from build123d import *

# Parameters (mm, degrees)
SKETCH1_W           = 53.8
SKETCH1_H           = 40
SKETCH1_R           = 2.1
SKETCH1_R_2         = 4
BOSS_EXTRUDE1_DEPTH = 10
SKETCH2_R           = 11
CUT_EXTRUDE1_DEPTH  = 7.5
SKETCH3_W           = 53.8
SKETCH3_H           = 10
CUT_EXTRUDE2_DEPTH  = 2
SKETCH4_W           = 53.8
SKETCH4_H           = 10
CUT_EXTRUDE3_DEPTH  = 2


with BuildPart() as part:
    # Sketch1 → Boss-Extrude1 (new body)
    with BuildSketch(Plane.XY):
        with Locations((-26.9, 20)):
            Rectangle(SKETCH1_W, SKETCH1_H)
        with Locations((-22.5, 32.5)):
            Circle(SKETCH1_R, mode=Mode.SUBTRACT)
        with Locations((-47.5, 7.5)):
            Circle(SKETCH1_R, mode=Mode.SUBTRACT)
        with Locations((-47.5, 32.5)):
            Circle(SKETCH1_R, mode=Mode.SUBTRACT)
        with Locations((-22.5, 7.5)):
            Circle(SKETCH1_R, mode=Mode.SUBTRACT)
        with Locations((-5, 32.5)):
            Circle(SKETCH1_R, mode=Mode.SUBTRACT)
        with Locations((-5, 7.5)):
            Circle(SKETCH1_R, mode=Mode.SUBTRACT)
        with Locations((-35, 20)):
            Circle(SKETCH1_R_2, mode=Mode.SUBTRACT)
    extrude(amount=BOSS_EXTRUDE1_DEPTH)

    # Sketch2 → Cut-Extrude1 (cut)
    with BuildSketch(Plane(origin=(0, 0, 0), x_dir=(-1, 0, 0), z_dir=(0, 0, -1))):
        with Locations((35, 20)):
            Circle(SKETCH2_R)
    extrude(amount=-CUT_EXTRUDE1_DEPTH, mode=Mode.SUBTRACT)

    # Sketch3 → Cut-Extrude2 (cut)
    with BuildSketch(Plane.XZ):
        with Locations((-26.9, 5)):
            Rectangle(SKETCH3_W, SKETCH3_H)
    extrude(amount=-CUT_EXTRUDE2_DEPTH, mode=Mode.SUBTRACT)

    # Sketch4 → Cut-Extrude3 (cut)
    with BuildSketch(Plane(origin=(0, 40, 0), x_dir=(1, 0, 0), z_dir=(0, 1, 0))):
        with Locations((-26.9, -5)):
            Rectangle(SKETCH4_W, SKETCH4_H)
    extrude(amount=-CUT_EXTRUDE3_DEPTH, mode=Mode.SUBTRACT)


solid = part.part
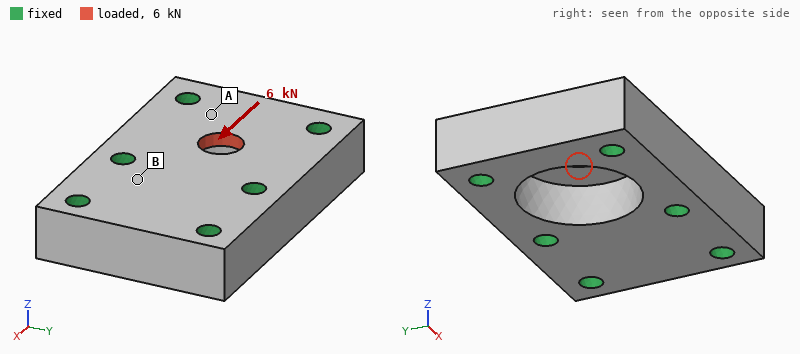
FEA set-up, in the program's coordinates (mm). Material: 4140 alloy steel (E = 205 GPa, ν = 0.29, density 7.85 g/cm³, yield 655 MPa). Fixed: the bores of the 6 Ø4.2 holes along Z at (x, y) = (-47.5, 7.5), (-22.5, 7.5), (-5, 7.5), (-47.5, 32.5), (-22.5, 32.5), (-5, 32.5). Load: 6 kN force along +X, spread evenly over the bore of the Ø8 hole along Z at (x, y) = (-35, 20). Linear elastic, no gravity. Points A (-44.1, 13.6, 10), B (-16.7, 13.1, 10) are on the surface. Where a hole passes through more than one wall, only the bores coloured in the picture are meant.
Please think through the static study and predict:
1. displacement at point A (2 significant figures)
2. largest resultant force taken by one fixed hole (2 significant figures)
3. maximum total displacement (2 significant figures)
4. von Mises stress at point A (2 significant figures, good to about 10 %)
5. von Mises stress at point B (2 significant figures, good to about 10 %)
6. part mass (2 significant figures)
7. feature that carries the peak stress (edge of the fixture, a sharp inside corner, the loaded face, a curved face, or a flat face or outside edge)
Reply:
1.9 µm
1.5 kN
5.0 µm
54 MPa
15 MPa
120 g
the loaded face
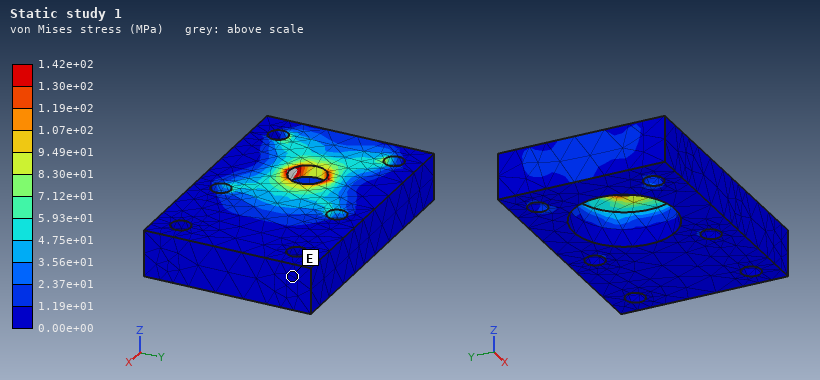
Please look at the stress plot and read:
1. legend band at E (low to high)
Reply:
0.00e+00 to 1.19e+01 MPa
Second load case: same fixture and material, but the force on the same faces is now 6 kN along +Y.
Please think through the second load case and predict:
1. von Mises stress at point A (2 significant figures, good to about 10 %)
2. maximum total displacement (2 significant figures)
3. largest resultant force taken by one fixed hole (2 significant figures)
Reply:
45 MPa
5.1 µm
1.6 kN
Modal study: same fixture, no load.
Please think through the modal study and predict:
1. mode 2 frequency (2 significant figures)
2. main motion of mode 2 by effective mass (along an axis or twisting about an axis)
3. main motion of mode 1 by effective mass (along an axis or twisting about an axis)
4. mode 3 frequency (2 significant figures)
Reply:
49 kHz
along Z
along Z
51 kHz
